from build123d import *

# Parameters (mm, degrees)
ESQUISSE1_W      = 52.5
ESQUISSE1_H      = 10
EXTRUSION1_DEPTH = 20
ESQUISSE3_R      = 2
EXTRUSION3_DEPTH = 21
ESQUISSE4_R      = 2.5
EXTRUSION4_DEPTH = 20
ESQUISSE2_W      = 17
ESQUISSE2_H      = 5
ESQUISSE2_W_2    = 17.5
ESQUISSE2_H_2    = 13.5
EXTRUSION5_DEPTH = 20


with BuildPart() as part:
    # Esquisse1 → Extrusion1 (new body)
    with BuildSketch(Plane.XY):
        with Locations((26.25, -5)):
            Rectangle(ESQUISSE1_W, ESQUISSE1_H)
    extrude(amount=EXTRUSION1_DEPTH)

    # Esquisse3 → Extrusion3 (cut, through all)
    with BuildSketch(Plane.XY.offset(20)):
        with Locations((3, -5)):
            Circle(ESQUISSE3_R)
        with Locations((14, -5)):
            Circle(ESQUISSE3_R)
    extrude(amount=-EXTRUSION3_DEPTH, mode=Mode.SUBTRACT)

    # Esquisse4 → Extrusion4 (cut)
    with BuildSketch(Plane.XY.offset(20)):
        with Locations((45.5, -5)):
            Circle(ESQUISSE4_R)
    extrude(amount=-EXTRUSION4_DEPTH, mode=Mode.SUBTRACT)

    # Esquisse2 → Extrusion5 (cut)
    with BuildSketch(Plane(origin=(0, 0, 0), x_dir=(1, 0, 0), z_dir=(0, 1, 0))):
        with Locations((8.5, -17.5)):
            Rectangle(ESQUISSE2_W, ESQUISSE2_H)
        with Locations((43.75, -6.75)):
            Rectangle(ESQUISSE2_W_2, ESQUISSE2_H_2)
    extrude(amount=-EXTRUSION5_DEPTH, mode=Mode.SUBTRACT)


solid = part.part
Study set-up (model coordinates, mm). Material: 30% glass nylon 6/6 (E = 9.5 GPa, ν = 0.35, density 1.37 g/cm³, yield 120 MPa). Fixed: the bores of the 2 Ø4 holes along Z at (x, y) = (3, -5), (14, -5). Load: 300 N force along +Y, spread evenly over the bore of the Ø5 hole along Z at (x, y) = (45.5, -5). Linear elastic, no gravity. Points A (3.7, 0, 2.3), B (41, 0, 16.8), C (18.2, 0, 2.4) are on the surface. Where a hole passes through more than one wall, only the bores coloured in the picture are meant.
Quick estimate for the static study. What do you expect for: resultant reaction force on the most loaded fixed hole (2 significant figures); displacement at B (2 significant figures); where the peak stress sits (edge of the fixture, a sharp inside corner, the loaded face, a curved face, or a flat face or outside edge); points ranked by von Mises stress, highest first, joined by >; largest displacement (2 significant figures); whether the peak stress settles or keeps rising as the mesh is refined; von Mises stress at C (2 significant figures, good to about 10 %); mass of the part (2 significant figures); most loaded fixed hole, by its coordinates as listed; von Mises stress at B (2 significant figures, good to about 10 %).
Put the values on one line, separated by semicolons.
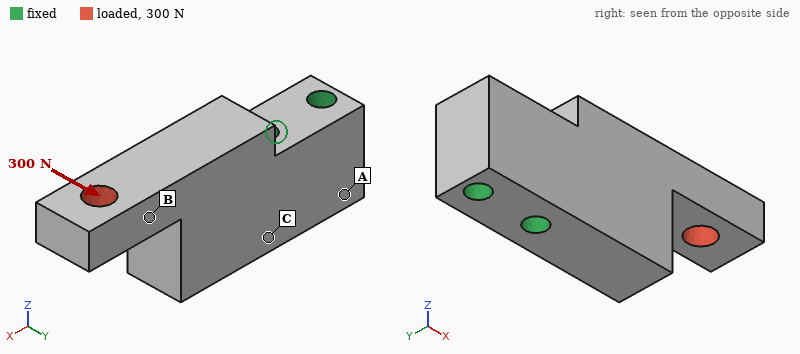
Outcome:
590 N; 0.32 mm; edge of the fixture; C > B > A; 0.55 mm; keeps rising; 27 MPa; 9.3 g; (14, -5); 17 MPa
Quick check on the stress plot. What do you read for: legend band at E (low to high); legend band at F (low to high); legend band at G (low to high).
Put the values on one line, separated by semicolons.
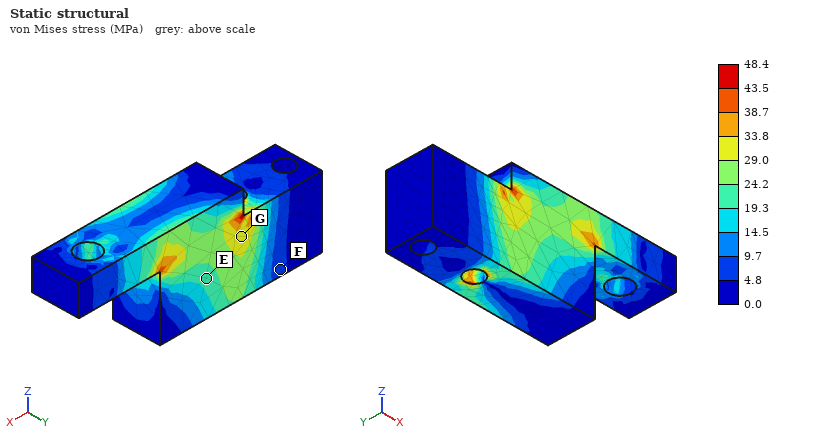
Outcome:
19.3 to 24.2 MPa; 4.8 to 9.7 MPa; 29.0 to 33.8 MPa
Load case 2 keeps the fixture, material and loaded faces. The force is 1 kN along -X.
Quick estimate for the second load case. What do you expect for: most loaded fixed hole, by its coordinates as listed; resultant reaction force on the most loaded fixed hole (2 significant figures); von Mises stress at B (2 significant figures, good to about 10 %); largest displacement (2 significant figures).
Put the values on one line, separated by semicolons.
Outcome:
(14, -5); 930 N; 18 MPa; 0.16 mm
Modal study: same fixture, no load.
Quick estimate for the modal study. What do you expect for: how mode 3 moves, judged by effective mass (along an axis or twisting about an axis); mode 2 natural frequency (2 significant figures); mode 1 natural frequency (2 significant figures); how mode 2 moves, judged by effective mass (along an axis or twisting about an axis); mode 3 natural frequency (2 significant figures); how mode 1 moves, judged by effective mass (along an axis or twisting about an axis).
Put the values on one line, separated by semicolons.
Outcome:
along Z; 4700 Hz; 3500 Hz; along Z; 11 kHz; along Y
